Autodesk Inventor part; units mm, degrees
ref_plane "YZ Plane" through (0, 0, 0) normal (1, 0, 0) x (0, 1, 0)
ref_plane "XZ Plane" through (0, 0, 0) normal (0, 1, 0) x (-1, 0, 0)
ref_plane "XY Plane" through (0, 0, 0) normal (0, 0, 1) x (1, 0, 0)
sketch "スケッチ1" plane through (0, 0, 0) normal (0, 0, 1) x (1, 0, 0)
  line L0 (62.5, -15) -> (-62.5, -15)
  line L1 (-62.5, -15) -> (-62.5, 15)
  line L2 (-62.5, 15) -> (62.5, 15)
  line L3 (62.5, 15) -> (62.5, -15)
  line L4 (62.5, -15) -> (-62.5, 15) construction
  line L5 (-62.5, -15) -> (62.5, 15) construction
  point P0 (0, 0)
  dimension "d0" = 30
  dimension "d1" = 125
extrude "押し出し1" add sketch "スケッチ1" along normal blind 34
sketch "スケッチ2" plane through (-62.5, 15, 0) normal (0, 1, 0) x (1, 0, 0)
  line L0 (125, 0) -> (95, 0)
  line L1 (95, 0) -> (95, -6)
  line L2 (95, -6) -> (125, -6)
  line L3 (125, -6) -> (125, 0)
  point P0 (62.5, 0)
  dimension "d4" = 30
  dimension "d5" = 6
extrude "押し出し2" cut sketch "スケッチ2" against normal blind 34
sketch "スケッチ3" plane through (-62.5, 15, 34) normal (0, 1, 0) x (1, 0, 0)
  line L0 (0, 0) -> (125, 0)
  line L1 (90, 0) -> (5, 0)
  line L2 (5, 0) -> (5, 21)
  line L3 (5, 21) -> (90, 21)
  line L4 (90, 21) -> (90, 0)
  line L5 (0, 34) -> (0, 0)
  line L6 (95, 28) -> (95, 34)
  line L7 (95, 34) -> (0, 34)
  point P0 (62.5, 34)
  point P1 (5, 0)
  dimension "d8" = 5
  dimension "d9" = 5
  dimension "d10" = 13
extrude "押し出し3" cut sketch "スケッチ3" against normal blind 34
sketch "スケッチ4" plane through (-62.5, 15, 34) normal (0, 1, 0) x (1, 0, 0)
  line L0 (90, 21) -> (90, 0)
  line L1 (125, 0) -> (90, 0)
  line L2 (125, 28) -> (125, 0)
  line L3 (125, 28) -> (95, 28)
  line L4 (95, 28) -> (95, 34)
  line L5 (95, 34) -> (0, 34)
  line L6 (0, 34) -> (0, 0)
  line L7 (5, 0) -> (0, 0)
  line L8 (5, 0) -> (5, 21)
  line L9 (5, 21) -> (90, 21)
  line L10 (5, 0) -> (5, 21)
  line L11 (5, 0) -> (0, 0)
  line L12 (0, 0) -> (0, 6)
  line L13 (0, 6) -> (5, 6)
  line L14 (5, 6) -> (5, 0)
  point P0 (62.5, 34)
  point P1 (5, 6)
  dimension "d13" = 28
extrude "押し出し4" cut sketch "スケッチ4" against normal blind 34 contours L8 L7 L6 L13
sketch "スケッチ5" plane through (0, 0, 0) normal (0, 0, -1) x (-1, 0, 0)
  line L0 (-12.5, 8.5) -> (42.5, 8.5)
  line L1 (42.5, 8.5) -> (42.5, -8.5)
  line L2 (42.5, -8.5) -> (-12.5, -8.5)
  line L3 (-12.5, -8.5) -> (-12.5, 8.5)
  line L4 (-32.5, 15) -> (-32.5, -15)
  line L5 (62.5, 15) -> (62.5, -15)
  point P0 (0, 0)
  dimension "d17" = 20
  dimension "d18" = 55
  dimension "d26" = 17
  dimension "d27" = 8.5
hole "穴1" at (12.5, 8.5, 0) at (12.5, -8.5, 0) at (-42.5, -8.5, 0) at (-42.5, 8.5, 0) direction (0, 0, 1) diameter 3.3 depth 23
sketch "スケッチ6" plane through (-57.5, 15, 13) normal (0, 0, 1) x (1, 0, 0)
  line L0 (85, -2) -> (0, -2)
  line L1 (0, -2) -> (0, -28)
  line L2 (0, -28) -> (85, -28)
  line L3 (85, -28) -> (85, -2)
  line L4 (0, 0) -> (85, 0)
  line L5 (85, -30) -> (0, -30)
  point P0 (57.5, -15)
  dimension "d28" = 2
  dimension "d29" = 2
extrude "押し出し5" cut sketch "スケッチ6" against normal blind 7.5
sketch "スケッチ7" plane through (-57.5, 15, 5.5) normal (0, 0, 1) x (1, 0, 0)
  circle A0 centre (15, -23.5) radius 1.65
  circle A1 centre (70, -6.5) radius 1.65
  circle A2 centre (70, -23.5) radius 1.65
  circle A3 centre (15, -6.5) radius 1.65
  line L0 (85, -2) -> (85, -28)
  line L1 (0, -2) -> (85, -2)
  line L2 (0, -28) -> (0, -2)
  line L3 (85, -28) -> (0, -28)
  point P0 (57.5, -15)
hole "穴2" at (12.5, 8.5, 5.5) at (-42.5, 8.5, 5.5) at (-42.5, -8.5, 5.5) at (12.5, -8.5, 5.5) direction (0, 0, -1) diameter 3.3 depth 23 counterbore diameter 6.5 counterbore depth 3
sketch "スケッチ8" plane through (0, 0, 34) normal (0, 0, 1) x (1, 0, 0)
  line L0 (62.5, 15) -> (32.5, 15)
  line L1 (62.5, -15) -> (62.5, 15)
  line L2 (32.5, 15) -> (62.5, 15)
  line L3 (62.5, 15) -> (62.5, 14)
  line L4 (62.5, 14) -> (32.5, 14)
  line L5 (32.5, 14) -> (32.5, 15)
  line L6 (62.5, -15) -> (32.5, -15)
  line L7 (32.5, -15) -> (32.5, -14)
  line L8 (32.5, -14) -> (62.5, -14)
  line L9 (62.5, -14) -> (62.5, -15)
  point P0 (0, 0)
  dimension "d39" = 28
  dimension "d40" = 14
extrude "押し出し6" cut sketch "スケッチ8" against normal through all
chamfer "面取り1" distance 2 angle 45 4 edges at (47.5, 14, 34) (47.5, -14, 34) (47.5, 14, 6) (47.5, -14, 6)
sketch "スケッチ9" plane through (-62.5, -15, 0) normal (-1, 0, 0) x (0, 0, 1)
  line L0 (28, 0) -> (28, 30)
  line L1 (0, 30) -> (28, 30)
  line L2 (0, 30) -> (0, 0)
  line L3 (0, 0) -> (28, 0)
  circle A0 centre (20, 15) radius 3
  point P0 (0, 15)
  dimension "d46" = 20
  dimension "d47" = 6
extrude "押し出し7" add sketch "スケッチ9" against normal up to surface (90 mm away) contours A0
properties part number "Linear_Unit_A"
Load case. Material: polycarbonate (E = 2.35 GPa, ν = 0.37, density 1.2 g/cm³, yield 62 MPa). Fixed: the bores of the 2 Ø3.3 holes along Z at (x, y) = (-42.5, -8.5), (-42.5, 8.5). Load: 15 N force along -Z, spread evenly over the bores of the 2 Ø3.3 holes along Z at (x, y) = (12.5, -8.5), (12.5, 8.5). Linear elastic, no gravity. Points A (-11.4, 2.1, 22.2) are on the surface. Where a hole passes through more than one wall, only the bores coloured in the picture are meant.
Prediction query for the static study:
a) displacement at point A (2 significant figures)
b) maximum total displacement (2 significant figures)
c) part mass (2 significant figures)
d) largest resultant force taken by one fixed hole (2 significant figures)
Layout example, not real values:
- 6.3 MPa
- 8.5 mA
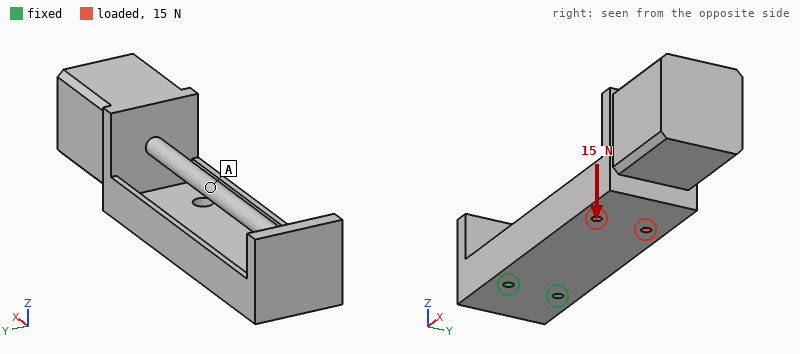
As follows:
- 0.47 mm
- 1.4 mm
- 61 g
- 7.7 N
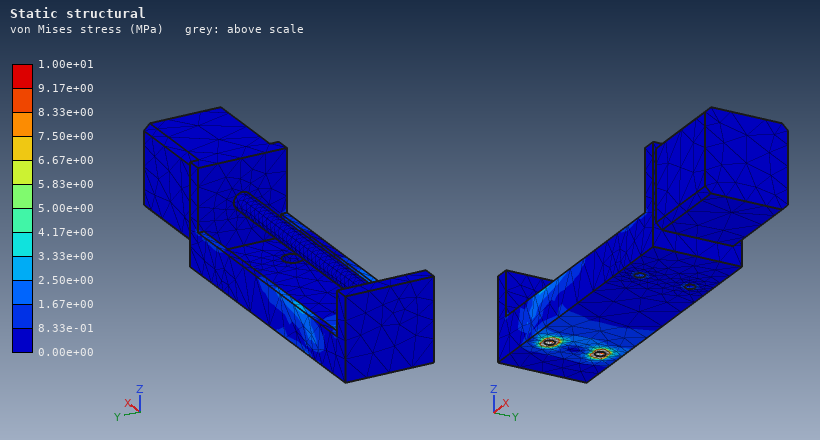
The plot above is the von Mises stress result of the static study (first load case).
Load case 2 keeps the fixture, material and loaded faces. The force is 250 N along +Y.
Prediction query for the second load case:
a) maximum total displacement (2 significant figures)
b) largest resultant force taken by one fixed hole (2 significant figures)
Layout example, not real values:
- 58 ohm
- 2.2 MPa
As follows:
- 1.5 mm
- 750 N
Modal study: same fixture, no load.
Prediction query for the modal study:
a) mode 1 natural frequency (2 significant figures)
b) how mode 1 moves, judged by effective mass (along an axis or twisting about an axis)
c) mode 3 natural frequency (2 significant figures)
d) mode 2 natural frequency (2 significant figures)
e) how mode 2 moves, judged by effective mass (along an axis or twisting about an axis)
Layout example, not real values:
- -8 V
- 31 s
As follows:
- 73 Hz
- along Z
- 490 Hz
- 180 Hz
- along Y
